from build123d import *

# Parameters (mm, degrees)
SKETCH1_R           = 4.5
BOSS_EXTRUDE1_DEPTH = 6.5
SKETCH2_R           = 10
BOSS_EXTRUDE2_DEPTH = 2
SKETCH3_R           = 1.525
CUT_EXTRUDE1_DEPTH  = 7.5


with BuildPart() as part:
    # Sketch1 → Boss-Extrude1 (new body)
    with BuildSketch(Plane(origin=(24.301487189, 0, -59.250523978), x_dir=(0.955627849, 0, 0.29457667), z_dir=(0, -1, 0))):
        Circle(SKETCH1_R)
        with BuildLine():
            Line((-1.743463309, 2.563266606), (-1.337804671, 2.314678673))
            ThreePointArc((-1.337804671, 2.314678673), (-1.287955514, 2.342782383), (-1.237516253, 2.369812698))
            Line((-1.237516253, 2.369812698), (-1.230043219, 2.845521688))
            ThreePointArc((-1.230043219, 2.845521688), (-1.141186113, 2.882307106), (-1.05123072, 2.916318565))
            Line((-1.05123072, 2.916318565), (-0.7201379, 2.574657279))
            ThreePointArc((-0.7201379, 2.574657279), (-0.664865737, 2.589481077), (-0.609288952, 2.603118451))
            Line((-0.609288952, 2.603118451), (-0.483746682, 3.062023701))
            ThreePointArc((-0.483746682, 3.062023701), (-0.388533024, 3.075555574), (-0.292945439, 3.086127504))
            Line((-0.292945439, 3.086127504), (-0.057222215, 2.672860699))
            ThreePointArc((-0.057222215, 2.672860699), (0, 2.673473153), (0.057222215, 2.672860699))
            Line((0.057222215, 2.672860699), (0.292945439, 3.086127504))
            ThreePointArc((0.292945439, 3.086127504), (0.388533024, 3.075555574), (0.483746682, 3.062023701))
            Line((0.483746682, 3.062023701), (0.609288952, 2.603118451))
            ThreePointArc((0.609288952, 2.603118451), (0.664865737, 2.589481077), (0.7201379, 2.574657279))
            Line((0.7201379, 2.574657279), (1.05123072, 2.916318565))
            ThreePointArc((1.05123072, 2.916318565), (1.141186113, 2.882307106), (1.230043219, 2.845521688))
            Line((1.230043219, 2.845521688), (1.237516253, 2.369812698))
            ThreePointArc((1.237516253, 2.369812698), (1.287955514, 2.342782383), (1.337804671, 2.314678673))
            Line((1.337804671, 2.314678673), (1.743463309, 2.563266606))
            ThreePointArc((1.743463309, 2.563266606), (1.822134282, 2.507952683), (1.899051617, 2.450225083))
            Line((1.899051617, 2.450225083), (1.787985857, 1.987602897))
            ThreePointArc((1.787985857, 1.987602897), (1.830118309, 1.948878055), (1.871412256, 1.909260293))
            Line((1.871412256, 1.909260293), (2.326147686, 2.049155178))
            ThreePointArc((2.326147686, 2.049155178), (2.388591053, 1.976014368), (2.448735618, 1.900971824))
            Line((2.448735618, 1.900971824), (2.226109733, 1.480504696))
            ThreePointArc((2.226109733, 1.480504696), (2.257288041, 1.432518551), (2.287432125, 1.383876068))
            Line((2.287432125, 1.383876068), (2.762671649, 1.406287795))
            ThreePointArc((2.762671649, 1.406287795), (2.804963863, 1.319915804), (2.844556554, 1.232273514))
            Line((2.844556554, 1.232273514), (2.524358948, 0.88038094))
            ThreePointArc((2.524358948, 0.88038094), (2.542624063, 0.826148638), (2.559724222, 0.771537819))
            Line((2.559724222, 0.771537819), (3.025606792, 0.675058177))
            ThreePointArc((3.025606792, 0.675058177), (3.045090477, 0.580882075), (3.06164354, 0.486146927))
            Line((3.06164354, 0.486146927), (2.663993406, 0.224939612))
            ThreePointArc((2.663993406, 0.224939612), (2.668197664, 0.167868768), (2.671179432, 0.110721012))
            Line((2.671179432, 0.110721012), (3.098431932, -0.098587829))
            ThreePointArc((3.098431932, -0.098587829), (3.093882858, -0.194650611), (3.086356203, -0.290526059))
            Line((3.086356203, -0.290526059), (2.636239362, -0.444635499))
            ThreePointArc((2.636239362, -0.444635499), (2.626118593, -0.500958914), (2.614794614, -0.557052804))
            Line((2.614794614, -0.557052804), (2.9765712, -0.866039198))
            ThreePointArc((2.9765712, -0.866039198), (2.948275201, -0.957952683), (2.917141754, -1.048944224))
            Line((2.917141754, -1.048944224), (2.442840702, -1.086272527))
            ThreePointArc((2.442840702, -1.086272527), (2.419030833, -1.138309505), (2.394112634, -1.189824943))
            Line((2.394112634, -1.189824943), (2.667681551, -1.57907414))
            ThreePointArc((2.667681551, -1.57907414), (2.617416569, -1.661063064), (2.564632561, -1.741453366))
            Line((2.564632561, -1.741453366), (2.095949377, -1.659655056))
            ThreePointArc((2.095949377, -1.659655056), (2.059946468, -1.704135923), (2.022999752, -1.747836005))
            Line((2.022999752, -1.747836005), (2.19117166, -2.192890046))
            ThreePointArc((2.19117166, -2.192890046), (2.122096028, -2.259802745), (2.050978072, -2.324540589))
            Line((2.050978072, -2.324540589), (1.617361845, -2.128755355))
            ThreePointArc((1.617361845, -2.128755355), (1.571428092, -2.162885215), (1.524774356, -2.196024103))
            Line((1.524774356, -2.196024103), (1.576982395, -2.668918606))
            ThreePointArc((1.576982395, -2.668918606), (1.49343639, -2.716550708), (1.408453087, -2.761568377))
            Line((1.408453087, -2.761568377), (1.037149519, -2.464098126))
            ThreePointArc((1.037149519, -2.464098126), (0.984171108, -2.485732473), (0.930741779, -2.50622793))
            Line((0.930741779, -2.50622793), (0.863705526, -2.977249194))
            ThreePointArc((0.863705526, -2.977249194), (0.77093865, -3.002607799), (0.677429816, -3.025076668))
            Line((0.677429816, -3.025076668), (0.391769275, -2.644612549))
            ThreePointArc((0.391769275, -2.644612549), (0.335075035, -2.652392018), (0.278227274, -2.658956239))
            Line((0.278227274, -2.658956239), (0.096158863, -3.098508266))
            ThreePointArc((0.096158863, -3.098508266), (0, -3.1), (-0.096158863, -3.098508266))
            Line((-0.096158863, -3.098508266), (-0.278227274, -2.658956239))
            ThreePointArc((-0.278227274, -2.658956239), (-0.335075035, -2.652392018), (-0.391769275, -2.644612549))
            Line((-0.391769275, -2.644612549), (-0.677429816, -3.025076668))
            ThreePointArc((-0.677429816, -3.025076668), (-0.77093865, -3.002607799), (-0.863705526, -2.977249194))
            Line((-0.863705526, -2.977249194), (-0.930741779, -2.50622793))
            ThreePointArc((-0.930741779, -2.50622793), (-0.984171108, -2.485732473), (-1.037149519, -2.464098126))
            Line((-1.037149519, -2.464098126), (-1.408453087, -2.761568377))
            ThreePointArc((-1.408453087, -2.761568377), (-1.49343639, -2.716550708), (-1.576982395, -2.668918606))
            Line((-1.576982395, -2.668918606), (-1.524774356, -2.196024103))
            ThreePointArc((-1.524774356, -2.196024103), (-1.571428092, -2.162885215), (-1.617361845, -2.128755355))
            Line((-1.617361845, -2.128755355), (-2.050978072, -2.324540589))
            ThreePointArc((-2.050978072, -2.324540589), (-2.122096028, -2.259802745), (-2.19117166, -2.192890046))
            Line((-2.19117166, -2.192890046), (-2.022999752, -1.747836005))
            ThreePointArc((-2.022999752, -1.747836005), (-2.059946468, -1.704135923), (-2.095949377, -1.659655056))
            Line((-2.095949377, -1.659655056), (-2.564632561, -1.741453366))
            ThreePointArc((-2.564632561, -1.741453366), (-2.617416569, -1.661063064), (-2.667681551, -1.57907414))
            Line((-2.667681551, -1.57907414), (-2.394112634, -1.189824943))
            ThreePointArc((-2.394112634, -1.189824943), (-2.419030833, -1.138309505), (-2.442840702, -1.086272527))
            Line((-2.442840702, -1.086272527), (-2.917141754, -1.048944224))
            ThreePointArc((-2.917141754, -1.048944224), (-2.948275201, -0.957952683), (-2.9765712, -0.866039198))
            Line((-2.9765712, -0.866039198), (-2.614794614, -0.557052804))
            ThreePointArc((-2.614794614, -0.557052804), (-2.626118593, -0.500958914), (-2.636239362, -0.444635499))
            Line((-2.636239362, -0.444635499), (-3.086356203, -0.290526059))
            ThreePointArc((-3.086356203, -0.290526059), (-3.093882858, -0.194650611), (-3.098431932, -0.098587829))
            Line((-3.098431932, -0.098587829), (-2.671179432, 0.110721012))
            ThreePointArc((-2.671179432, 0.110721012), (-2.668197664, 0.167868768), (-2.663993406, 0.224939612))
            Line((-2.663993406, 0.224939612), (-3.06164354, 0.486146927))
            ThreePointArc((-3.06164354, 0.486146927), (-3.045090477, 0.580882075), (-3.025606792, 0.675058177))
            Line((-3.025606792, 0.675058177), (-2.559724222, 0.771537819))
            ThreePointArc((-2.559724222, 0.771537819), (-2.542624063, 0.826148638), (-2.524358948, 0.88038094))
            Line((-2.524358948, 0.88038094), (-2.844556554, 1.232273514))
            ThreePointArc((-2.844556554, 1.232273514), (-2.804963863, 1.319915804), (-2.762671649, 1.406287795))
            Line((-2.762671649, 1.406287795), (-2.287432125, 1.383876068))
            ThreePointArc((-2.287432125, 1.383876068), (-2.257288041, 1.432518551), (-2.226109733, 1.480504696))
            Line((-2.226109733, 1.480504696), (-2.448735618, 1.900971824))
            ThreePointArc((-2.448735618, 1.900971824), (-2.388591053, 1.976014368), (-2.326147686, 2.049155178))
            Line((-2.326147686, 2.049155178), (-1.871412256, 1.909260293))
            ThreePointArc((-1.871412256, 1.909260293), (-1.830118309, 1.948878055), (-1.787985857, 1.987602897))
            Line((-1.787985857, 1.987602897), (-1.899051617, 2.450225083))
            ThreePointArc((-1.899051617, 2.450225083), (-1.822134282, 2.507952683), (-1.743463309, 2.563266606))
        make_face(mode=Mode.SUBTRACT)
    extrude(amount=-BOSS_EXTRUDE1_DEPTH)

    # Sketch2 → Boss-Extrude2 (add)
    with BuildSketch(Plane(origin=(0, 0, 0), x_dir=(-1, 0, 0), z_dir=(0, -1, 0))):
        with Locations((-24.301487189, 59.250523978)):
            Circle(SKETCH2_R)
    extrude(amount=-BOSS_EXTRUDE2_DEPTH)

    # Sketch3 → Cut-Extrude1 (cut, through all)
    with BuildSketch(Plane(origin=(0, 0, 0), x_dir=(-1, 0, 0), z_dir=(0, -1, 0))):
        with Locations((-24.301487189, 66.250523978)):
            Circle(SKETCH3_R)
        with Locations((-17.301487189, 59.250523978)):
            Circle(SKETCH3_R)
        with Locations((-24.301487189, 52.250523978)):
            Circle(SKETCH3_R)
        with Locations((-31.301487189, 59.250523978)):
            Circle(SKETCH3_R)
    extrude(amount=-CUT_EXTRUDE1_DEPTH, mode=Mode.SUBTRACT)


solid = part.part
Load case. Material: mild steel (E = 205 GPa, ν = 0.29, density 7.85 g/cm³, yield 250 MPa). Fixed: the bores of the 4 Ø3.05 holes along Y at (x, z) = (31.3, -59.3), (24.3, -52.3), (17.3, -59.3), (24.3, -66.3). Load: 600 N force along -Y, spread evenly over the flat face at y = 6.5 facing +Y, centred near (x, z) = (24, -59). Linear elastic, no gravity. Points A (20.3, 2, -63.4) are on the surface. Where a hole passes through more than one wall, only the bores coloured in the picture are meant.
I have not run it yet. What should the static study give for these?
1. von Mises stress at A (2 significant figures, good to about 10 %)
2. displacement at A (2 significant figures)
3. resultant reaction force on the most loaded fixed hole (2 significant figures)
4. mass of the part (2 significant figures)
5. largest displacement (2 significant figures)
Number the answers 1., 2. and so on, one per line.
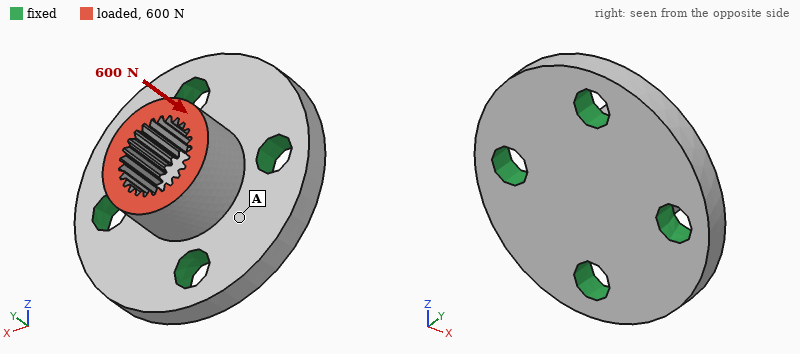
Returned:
1. 10.0 MPa
2. 0.35 µm
3. 160 N
4. 5.8 g
5. 1.00 µm
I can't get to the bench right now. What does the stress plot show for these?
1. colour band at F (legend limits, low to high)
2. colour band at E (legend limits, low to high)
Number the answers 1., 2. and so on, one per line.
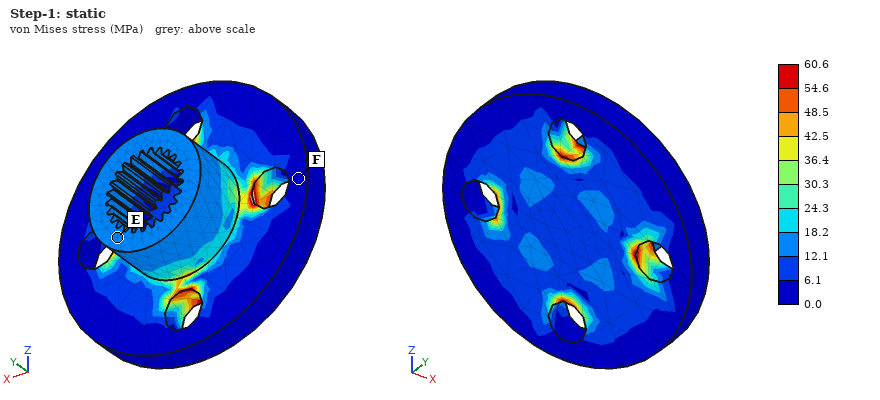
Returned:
1. 0.0 to 6.1 MPa
2. 12.1 to 18.2 MPa
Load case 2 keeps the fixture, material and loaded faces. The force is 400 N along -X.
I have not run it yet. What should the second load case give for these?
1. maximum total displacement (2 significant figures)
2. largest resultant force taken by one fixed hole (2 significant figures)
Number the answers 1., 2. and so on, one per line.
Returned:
1. 3.2 µm
2. 220 N
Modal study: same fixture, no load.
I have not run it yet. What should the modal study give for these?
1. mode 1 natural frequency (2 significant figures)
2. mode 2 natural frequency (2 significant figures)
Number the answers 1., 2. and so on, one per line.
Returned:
1. 78 kHz
2. 78 kHz
